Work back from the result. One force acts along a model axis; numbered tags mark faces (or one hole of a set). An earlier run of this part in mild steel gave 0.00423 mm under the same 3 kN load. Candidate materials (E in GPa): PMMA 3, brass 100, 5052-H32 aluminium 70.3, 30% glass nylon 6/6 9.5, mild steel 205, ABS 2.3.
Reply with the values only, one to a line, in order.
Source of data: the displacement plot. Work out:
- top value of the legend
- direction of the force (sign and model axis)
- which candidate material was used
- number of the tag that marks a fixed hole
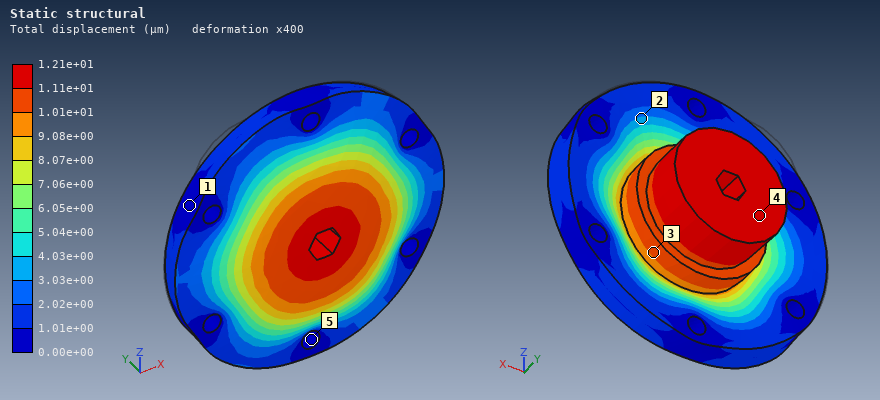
1.21e+01 µm
-Y
5052-H32 aluminium
5
